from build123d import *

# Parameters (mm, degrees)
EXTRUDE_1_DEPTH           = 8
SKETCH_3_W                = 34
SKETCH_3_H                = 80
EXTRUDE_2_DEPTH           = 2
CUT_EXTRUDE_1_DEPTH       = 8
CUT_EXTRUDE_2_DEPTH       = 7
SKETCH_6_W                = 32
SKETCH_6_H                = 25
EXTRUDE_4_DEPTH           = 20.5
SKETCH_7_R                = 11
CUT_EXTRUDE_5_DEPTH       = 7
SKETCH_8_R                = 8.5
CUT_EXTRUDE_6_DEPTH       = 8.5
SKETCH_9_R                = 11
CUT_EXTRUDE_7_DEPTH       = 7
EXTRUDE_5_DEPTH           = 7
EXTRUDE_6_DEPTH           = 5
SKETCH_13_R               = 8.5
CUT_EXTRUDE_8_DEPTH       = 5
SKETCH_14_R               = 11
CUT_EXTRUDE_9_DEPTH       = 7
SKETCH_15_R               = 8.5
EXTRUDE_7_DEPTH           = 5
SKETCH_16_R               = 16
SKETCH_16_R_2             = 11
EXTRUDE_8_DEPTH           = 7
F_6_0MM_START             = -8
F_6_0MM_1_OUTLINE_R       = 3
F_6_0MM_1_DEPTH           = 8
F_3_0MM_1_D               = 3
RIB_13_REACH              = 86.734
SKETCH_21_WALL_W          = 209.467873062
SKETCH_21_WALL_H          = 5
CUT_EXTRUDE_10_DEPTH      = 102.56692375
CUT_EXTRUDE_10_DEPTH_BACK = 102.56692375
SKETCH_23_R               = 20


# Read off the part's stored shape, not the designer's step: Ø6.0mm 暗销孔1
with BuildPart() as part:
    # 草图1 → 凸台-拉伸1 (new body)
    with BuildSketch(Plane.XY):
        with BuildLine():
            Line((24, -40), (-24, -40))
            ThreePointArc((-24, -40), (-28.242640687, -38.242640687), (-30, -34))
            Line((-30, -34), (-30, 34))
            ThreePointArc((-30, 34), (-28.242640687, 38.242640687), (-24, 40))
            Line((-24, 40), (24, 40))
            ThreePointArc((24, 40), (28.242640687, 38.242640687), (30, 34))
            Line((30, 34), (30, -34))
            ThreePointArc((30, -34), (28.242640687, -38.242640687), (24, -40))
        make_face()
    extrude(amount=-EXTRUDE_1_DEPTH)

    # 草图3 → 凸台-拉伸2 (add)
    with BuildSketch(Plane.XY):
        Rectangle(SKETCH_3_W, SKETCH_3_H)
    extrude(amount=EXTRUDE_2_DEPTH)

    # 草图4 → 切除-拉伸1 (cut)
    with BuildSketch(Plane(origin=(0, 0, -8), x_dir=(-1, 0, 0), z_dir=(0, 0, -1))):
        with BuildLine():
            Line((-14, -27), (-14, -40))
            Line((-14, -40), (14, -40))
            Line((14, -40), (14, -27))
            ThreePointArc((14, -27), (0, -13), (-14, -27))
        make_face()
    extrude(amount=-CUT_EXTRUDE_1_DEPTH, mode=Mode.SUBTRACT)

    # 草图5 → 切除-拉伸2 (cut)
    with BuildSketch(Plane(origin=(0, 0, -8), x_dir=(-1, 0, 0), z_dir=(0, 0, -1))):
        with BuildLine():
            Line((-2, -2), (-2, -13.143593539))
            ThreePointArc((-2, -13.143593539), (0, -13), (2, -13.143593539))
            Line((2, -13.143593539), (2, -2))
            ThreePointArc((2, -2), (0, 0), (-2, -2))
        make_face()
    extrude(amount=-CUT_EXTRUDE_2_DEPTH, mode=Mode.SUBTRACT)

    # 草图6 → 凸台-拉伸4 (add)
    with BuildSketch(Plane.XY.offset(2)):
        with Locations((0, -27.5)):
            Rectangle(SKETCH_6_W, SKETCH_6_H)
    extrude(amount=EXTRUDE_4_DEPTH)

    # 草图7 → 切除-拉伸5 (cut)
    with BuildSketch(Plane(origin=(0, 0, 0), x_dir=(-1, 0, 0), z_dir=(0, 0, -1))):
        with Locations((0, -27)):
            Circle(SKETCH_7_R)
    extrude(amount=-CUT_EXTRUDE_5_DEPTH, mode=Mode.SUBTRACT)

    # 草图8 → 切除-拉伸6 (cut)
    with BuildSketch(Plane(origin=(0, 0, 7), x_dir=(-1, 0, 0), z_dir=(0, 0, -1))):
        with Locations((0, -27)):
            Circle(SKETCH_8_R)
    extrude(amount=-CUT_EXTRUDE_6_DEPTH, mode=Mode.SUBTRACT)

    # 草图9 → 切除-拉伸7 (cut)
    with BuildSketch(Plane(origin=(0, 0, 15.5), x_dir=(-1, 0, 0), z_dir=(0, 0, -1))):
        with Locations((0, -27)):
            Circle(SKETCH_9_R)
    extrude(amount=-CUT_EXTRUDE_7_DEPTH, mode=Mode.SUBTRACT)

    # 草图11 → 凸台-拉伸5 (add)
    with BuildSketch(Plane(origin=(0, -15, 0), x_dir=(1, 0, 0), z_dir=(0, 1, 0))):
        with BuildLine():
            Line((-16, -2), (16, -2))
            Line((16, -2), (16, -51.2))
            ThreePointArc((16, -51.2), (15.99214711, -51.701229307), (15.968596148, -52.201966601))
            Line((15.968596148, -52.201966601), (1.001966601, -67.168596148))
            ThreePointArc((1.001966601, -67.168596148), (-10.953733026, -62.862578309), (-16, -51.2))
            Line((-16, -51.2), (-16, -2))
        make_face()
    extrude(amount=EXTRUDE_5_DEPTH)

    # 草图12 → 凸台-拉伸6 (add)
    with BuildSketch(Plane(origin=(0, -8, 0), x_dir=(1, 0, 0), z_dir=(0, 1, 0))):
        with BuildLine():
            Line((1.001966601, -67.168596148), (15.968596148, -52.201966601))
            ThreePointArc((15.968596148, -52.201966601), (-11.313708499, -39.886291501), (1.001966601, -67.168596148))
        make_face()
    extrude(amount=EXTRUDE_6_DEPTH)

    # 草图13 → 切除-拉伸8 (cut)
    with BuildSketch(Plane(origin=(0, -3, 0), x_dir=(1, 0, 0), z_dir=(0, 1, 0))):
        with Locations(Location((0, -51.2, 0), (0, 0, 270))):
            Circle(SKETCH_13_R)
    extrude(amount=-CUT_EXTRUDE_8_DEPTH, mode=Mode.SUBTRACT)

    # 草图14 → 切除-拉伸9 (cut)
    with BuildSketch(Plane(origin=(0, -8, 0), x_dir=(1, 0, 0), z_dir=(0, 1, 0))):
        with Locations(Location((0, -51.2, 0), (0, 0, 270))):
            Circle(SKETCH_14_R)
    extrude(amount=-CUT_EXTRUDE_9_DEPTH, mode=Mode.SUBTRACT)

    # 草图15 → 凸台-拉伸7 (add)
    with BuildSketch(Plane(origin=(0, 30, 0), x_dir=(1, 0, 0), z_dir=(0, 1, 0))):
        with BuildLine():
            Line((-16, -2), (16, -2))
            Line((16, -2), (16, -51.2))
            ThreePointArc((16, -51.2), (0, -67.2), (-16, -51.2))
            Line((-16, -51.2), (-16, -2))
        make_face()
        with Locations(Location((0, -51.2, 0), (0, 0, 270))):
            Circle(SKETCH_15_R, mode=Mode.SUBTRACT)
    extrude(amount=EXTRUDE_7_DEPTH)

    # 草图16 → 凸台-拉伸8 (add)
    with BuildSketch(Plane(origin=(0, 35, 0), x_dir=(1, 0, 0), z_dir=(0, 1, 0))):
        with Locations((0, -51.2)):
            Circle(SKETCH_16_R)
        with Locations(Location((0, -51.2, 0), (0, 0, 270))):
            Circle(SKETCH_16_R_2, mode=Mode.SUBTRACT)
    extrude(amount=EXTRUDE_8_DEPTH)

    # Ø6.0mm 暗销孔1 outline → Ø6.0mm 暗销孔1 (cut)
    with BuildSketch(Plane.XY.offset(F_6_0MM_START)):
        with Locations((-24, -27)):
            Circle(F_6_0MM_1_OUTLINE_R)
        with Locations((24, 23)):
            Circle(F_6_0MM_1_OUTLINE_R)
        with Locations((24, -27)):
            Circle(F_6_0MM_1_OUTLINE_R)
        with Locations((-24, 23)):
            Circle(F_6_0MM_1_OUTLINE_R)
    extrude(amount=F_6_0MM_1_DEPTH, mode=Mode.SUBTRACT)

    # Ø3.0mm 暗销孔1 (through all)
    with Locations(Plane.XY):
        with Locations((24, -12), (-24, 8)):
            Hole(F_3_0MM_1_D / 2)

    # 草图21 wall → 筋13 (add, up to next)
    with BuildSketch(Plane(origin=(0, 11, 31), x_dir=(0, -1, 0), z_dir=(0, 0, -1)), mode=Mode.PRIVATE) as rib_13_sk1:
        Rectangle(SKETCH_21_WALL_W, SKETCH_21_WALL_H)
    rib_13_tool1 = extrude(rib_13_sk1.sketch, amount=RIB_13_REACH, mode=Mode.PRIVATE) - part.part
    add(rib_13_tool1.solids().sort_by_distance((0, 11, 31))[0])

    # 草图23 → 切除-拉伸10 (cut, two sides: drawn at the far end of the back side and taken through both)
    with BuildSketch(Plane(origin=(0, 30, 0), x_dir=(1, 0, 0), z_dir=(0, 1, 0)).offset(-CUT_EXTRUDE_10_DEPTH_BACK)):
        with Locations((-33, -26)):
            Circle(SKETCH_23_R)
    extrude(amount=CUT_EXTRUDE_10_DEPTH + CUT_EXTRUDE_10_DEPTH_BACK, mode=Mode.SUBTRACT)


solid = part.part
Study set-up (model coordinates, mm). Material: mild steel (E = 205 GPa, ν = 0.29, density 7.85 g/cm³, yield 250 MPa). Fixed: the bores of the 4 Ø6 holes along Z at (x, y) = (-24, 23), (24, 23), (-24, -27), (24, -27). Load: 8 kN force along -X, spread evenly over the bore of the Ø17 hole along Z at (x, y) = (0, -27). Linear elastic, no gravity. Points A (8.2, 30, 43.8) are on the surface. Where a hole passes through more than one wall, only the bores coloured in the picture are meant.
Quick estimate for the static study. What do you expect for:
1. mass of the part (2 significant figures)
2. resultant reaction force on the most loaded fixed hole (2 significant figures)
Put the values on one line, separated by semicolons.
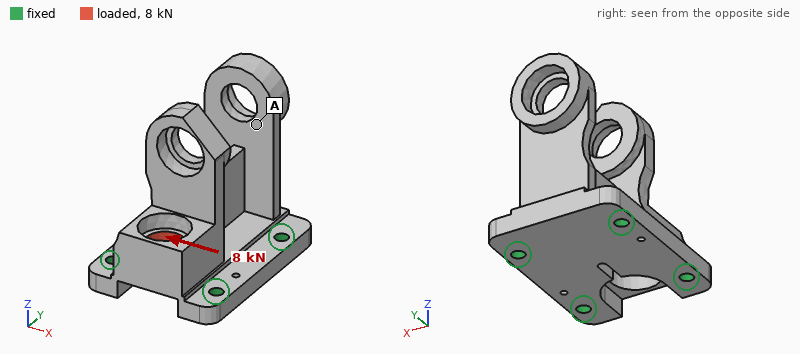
590 g; 4.2 kN
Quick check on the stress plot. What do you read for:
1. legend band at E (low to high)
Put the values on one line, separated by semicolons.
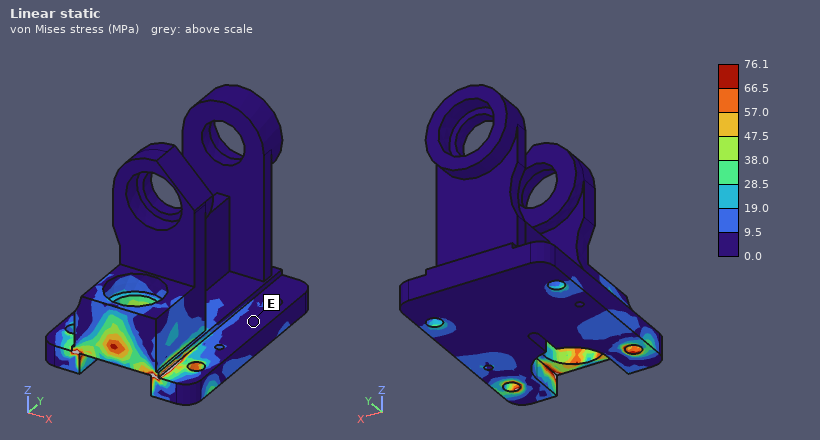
0.0 to 9.5 MPa
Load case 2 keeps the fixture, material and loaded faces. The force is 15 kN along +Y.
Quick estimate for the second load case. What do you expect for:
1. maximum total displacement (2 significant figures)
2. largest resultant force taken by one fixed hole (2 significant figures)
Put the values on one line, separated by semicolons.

28 µm; 4.9 kN
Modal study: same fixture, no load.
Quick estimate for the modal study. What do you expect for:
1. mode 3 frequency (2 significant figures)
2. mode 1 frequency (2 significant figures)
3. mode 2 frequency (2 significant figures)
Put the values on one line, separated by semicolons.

3400 Hz; 2100 Hz; 3400 Hz
